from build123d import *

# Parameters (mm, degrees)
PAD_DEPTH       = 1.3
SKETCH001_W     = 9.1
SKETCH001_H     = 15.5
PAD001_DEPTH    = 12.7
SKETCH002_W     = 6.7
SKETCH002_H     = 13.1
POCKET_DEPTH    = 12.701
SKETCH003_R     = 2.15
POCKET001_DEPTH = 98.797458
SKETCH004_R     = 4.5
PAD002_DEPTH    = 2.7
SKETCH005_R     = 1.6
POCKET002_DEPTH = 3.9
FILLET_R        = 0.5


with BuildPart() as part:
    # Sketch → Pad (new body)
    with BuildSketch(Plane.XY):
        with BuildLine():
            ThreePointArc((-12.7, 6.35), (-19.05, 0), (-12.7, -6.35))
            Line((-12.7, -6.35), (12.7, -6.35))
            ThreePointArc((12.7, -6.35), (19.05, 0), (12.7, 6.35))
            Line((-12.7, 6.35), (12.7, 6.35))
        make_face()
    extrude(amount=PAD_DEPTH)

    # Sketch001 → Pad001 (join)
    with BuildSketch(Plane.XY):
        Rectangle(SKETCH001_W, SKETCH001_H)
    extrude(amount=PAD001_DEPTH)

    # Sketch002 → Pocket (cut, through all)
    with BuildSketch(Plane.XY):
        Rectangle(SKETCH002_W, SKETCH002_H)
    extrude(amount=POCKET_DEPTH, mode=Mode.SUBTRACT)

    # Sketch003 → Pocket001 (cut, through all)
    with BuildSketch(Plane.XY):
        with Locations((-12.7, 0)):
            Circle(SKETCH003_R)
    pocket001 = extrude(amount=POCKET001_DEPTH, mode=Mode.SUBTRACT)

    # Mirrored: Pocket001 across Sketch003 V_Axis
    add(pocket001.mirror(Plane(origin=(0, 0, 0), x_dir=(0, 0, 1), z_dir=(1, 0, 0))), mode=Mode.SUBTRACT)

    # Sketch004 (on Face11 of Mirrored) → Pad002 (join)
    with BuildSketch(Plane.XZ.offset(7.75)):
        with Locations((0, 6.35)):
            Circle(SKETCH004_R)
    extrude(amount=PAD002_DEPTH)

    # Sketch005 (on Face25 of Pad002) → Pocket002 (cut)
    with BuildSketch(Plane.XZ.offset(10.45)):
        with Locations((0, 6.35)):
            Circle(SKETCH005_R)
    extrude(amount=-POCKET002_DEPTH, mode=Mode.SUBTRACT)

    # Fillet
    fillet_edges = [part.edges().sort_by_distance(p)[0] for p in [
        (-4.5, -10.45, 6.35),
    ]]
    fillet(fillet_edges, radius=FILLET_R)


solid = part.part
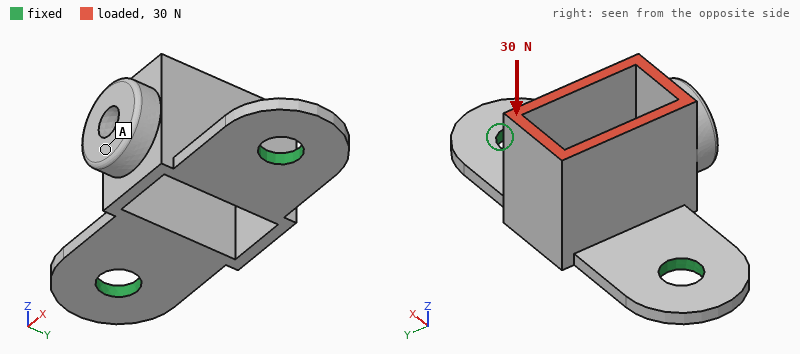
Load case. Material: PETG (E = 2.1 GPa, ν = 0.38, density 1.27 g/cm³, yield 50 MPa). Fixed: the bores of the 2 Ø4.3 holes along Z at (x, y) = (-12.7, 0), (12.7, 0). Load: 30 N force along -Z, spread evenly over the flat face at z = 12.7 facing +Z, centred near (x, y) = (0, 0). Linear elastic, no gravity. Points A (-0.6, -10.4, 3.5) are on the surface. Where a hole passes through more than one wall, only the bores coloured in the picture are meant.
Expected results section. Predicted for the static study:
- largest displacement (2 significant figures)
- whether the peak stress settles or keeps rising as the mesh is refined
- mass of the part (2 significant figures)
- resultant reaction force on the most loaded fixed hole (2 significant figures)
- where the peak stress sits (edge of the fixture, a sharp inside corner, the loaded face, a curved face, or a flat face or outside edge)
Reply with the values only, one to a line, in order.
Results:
0.17 mm
keeps rising
1.5 g
17 N
edge of the fixture
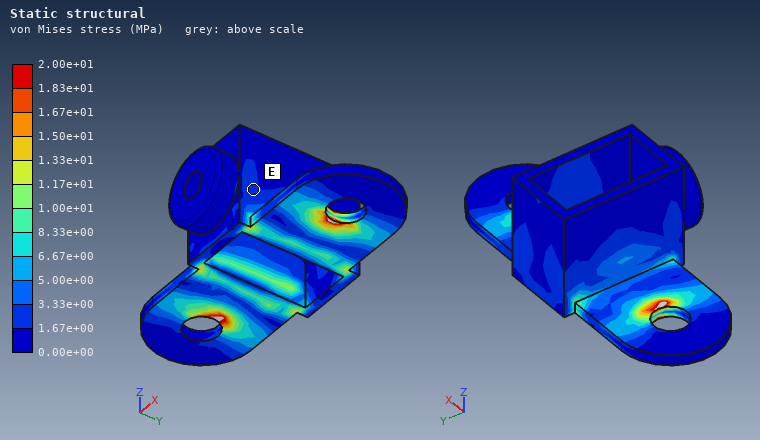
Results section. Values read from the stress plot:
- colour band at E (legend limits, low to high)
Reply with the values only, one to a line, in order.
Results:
1.67e+00 to 3.33e+00 MPa
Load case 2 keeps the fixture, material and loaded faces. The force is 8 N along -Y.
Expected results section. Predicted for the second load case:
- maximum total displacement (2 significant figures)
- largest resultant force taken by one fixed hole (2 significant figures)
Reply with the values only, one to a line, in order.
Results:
0.43 mm
4.0 N
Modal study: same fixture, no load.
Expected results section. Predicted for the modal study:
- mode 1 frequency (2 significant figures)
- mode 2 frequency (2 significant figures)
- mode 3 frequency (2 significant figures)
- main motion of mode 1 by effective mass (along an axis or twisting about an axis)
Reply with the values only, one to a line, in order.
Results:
960 Hz
2100 Hz
2200 Hz
along Y
